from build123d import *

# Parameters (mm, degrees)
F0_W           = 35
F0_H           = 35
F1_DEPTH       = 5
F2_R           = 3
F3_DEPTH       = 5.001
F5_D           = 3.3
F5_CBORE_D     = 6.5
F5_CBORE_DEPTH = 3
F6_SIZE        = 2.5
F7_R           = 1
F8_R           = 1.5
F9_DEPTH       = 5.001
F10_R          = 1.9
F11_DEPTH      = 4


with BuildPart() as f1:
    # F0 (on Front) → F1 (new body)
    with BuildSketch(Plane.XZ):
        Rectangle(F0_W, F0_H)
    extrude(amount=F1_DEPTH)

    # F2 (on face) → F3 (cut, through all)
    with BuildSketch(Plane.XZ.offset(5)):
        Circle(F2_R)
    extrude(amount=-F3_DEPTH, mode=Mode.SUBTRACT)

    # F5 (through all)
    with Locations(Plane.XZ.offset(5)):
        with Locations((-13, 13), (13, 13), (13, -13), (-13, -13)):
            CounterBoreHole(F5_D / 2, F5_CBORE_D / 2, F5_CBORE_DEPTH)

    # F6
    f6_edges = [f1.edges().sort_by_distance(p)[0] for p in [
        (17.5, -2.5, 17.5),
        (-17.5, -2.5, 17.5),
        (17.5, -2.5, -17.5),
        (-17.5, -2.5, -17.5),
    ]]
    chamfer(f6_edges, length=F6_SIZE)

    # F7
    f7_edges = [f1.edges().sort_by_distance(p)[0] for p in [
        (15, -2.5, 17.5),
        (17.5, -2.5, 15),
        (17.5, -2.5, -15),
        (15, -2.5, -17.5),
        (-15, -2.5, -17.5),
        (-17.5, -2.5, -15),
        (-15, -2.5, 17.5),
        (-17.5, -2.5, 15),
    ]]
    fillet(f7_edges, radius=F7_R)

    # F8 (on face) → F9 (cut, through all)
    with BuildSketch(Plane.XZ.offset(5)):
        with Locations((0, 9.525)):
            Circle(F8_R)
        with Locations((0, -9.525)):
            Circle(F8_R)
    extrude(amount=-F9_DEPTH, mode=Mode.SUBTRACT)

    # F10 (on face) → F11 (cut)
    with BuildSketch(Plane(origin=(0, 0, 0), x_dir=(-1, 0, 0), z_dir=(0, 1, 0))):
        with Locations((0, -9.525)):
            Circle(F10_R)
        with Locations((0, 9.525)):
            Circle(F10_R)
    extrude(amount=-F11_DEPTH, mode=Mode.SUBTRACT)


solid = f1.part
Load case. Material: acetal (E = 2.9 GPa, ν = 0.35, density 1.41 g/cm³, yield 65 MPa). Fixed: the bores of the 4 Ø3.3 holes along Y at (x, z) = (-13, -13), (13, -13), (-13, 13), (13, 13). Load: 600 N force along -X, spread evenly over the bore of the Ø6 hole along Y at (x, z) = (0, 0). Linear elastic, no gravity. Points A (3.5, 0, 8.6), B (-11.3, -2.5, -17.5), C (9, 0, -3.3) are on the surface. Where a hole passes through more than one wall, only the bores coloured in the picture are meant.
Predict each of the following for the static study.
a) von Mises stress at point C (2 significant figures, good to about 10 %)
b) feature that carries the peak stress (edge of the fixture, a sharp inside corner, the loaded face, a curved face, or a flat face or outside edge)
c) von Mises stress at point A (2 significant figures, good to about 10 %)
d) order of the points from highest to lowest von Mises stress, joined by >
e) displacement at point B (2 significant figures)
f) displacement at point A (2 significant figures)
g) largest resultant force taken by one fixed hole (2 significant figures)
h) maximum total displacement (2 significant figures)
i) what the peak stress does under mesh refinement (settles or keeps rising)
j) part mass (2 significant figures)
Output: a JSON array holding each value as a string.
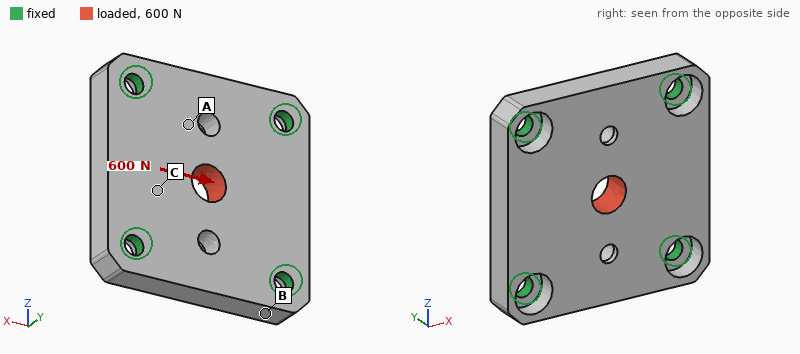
["3.6 MPa", "edge of the fixture", "4.9 MPa", "A > C > B", "7.1 µm", "21 µm", "160 N", "40 µm", "keeps rising", "7.5 g"]
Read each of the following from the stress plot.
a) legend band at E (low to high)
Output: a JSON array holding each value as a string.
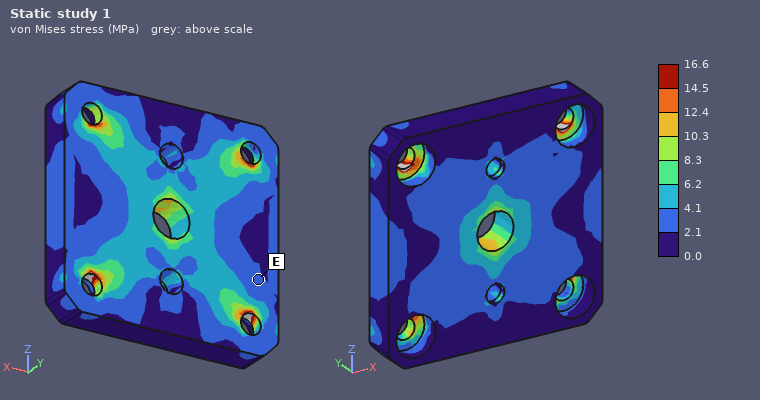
["2.1 to 4.1 MPa"]
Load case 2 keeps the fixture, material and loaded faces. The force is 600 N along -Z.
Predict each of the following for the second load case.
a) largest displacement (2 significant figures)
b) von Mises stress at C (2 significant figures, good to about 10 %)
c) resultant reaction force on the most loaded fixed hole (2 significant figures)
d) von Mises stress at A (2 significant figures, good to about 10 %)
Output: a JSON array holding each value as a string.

["41 µm", "3.3 MPa", "160 N", "3.9 MPa"]
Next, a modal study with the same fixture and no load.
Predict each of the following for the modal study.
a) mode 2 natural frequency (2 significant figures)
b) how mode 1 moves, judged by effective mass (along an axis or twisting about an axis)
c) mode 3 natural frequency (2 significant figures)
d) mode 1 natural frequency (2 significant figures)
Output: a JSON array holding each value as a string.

["7700 Hz", "along Y", "7700 Hz", "5300 Hz"]
